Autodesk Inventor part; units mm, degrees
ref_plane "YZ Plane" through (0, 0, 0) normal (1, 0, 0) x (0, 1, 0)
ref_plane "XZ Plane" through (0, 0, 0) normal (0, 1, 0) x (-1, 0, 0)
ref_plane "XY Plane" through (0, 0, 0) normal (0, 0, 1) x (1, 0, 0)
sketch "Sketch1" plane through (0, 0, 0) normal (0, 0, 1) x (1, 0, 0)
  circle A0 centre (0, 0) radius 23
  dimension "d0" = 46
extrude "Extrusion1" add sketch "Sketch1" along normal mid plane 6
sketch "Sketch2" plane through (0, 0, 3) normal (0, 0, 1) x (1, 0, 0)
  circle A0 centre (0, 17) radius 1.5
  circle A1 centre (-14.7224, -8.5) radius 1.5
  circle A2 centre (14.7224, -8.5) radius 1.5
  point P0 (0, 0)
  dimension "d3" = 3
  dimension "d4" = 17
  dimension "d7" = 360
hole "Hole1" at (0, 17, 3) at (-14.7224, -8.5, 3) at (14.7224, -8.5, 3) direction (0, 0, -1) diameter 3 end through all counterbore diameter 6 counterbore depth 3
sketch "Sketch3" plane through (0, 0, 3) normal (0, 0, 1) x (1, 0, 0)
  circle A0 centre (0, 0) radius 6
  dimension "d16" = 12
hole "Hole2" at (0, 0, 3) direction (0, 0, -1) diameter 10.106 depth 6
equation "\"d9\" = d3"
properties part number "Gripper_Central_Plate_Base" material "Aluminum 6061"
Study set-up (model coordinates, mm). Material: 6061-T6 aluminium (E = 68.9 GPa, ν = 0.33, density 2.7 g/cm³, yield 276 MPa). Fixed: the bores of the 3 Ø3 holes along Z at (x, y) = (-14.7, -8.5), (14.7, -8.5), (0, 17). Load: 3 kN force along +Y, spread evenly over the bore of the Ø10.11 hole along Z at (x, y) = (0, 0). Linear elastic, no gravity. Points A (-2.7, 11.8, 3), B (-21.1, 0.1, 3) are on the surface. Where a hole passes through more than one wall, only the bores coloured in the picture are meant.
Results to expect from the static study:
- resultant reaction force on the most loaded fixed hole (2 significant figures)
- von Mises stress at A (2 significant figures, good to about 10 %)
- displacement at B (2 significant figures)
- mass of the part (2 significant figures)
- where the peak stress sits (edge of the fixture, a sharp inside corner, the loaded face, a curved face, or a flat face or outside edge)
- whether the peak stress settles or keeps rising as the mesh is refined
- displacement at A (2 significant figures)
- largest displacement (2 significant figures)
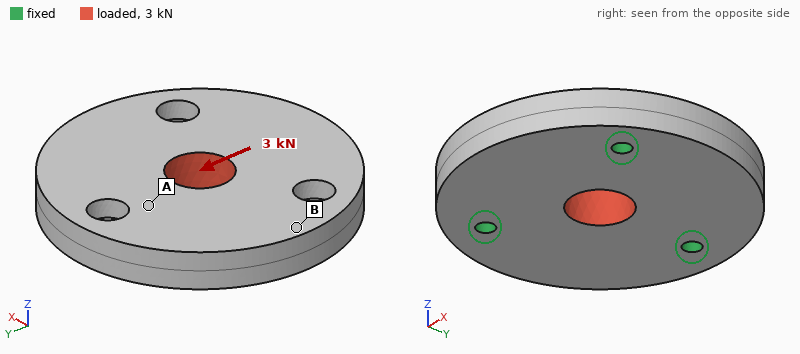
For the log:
1.1 kN
17 MPa
3.3 µm
25 g
edge of the fixture
keeps rising
3.0 µm
8.0 µm
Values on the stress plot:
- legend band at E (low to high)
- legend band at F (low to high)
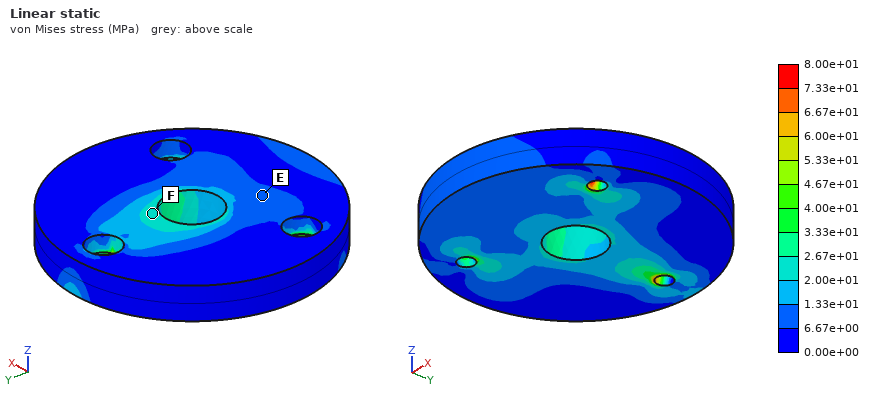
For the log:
6.67e+00 to 1.33e+01 MPa
2.00e+01 to 2.67e+01 MPa
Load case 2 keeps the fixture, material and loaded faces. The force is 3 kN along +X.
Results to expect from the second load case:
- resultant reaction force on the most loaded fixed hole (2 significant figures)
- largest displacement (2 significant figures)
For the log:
1.0 kN
6.9 µm
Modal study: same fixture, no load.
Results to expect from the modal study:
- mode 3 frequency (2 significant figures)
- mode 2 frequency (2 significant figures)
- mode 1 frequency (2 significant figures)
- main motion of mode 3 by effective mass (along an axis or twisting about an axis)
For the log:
17 kHz
12 kHz
12 kHz
along Z
